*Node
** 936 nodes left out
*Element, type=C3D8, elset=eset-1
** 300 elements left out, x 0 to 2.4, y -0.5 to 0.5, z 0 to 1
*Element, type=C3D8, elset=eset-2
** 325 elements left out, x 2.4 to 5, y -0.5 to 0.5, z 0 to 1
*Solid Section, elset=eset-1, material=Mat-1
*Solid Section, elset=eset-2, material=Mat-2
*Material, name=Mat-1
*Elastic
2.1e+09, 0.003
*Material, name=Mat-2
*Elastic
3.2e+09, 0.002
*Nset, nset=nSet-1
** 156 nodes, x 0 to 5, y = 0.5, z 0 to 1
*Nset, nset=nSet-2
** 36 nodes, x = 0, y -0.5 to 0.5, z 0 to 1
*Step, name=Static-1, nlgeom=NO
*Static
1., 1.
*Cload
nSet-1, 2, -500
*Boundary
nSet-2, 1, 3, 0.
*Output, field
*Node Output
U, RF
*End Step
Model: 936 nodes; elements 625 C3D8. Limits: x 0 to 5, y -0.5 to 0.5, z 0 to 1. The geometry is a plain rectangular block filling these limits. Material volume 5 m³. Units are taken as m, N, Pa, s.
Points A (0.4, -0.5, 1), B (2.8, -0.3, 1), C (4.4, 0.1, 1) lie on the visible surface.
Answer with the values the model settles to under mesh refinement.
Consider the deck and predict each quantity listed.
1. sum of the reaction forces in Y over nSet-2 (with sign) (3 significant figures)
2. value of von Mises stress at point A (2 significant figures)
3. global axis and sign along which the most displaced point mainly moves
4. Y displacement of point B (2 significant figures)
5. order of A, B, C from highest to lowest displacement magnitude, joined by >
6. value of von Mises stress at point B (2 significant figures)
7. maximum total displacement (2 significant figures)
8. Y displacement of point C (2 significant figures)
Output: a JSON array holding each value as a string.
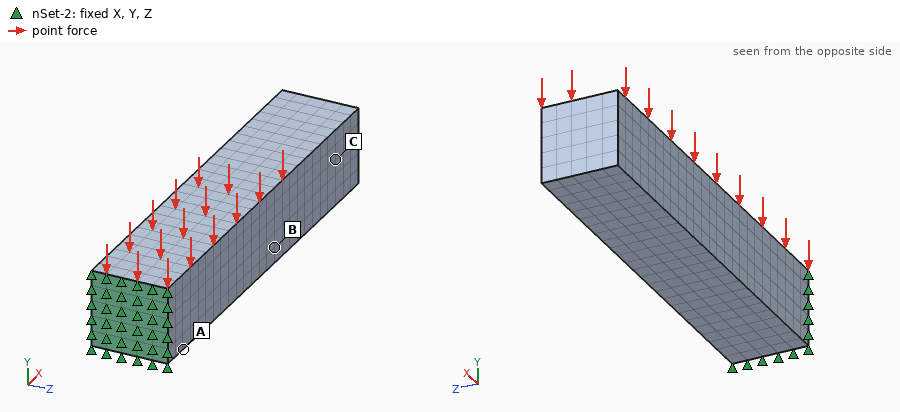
["78000 N", "9.9e+05 Pa", "-Y", "-0.0032 m", "C > B > A", "1.6e+05 Pa", "0.0071 m", "-0.0060 m"]
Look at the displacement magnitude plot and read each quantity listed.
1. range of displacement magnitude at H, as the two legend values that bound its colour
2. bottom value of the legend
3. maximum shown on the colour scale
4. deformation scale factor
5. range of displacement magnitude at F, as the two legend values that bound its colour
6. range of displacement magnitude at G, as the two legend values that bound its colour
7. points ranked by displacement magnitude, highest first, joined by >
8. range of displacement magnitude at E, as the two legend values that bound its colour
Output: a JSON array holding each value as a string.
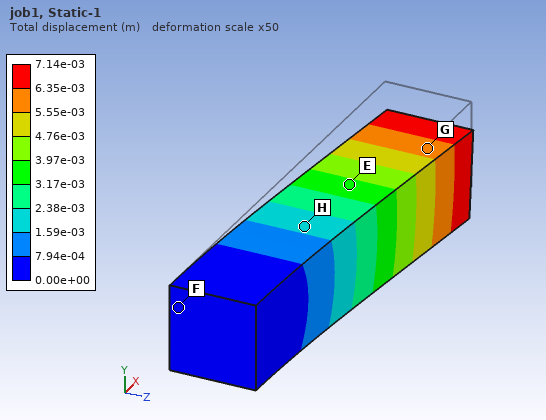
["1.59e-03 to 2.38e-03 m", "0.00e+00 m", "7.14e-03 m", "50", "0.00e+00 to 7.94e-04 m", "5.55e-03 to 6.35e-03 m", "G > E > H > F", "3.17e-03 to 3.97e-03 m"]
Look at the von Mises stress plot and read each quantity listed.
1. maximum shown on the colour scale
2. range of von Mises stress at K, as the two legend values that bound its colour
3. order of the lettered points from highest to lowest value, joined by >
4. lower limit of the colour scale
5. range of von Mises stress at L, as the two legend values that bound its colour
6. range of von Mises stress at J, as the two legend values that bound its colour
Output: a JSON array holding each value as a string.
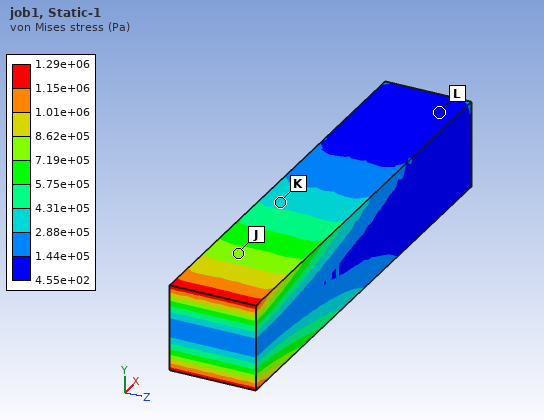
["1.29e+06 Pa", "2.88e+05 to 4.31e+05 Pa", "J > K > L", "4.55e+02 Pa", "4.55e+02 to 1.44e+05 Pa", "7.19e+05 to 8.62e+05 Pa"]
